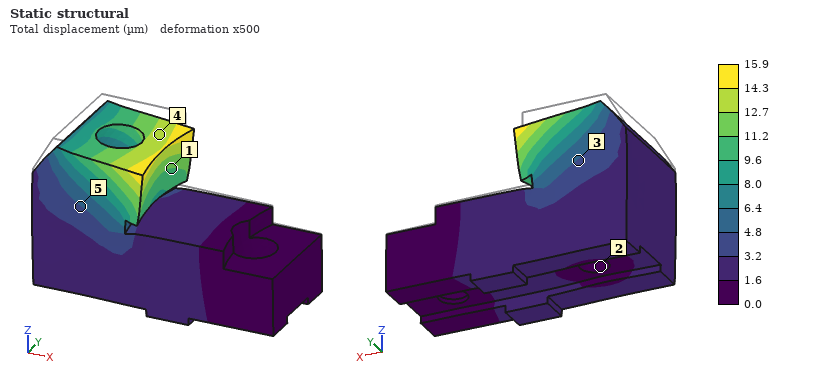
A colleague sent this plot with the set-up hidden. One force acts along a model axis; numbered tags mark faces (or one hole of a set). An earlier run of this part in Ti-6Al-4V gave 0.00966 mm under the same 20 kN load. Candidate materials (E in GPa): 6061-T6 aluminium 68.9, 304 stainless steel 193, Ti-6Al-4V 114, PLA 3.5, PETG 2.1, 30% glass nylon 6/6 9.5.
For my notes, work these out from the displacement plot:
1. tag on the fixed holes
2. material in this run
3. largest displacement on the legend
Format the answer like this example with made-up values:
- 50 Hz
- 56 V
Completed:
- 2
- 6061-T6 aluminium
- 15.9 µm
